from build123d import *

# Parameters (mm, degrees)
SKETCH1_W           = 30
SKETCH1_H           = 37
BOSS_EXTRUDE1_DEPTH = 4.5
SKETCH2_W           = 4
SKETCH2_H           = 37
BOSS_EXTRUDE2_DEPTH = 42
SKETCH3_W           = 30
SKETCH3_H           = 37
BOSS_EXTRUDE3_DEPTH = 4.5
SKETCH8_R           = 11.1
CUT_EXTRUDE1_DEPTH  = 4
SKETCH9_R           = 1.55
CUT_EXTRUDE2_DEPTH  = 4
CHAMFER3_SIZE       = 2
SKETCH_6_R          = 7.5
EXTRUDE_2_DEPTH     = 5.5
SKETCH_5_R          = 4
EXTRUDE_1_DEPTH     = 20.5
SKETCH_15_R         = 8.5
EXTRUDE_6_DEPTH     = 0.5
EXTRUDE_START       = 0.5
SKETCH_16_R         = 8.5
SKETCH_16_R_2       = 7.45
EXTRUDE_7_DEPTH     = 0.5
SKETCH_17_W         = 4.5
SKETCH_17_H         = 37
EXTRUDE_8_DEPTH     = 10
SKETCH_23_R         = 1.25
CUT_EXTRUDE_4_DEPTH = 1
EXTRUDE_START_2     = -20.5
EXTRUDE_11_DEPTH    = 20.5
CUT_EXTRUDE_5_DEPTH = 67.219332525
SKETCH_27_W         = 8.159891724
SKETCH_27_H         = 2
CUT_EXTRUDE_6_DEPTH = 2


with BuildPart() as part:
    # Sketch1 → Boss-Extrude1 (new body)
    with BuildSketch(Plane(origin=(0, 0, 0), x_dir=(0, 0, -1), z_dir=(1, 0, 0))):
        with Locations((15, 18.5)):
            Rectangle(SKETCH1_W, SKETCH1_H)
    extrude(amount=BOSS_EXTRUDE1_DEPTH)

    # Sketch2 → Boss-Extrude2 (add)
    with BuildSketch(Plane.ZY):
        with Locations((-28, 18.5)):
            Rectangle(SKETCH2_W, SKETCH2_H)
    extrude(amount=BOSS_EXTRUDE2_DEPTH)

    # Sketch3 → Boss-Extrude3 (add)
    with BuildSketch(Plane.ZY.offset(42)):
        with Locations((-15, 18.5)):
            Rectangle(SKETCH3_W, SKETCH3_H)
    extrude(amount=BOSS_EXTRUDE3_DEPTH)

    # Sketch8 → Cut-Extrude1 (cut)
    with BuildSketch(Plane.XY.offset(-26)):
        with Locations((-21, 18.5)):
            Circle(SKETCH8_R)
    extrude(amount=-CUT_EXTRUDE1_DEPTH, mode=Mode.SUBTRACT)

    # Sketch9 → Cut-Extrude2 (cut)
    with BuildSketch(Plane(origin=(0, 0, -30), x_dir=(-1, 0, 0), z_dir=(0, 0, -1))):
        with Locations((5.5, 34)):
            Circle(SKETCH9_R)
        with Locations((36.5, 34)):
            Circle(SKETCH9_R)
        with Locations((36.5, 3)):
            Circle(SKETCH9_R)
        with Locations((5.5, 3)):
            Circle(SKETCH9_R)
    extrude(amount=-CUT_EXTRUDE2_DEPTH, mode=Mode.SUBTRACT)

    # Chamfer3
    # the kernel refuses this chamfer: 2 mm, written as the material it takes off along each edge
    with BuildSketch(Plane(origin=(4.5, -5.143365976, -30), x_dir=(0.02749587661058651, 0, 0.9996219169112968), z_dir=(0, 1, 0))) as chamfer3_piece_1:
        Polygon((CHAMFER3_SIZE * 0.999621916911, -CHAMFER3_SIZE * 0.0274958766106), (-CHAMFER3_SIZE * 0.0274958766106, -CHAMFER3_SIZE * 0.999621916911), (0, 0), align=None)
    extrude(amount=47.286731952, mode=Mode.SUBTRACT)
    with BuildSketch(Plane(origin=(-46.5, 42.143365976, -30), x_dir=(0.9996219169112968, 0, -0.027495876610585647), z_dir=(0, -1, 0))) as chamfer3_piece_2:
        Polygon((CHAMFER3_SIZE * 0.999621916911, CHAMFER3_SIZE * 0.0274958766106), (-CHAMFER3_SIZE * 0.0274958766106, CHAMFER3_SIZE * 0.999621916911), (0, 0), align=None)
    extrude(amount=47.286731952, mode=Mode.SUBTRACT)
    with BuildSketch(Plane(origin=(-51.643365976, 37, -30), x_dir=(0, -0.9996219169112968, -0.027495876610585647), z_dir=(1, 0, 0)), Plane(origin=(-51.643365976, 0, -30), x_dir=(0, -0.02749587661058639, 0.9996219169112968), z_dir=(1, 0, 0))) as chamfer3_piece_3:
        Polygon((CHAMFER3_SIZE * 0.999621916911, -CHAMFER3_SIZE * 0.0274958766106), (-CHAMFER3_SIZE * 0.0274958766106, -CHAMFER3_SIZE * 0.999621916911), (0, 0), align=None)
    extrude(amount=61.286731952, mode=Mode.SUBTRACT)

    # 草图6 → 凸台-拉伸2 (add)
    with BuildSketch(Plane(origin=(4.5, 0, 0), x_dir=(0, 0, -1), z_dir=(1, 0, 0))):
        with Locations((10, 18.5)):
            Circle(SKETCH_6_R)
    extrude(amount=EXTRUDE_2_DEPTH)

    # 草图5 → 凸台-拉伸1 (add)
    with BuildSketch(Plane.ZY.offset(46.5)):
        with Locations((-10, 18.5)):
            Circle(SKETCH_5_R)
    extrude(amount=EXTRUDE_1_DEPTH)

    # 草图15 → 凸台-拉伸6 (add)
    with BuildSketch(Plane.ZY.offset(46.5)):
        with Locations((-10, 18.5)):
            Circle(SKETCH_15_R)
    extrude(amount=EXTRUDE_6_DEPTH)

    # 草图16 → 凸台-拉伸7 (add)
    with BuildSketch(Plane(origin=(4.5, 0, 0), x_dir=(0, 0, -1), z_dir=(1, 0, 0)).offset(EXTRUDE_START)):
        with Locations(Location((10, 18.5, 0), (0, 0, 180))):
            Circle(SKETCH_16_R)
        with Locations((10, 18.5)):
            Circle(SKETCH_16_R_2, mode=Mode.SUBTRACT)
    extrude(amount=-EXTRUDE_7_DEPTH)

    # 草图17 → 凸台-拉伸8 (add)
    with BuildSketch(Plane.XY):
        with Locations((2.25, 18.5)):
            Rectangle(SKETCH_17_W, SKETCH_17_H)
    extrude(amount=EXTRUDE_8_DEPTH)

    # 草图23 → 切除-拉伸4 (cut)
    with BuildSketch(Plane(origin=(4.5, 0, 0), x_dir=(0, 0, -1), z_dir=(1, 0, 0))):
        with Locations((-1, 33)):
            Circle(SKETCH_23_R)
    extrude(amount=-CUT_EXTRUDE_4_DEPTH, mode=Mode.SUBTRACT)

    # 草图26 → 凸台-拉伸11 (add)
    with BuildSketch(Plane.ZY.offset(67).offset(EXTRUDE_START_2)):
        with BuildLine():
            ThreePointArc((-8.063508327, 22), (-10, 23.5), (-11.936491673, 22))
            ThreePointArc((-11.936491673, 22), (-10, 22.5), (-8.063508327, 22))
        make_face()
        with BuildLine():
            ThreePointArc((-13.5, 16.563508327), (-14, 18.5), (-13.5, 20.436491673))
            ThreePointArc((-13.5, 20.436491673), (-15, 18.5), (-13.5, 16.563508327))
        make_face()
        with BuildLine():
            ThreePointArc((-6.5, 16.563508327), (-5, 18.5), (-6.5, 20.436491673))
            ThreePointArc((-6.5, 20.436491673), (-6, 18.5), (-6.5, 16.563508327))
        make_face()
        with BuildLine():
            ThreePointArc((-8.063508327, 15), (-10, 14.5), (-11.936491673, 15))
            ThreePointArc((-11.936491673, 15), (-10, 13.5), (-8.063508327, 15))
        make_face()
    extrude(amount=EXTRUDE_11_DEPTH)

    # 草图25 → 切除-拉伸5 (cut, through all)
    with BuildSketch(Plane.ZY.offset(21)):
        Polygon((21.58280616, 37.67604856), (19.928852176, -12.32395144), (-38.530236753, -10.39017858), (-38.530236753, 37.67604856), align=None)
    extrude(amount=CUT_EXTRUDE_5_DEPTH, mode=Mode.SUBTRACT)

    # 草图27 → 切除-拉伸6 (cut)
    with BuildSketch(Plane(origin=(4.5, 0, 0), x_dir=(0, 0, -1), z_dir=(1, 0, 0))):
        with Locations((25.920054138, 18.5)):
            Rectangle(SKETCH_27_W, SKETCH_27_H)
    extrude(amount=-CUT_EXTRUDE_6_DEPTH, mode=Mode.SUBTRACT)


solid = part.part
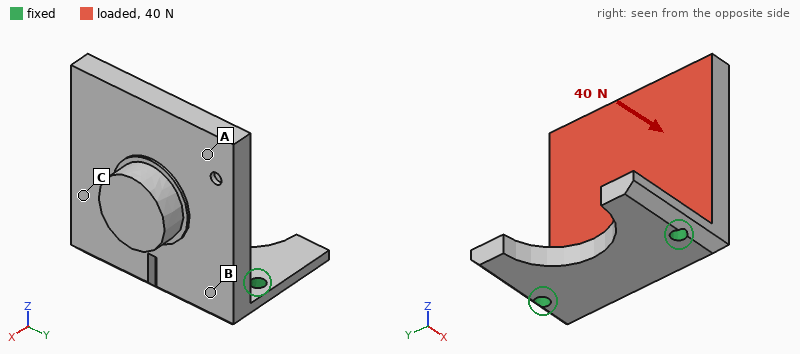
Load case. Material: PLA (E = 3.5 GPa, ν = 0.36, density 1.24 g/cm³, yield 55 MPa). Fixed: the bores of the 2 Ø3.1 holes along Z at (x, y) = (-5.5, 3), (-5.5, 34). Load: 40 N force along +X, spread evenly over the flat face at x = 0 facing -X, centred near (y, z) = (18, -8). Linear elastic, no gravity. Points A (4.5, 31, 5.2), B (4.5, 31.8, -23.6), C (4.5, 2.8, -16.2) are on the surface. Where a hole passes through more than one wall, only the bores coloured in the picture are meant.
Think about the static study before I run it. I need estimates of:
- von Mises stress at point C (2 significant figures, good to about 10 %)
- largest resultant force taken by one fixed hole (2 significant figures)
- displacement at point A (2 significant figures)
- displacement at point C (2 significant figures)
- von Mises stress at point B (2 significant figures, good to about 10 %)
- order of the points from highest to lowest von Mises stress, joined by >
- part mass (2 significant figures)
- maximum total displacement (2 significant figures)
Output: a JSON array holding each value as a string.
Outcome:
["2.9 MPa", "23 N", "0.57 mm", "0.19 mm", "4.6 MPa", "B > C > A", "12 g", "0.66 mm"]
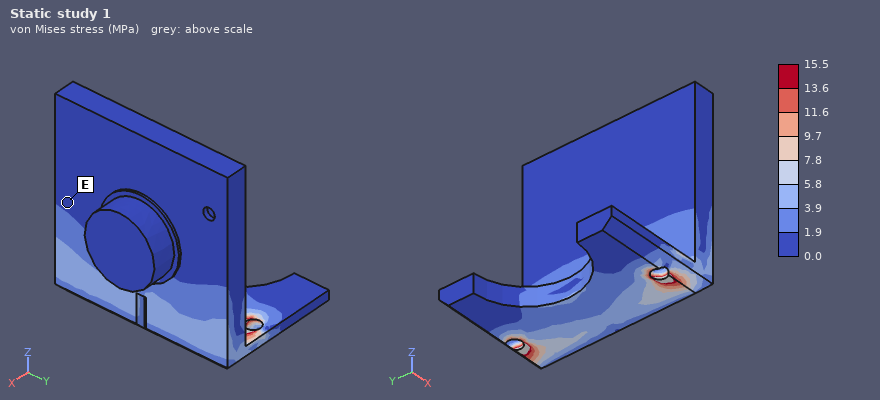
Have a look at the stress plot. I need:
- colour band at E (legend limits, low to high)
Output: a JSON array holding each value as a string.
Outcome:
["0.0 to 1.9 MPa"]
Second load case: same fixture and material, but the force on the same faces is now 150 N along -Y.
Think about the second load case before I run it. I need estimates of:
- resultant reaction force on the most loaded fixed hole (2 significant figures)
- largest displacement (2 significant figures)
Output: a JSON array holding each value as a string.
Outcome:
["130 N", "0.24 mm"]
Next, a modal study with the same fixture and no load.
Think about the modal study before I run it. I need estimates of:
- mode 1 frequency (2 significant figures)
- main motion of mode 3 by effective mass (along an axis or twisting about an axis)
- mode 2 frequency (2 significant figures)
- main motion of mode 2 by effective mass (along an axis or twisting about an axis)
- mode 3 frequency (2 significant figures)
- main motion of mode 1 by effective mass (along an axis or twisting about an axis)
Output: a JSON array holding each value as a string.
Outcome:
["530 Hz", "along Y", "1700 Hz", "along Y", "2400 Hz", "along X"]
